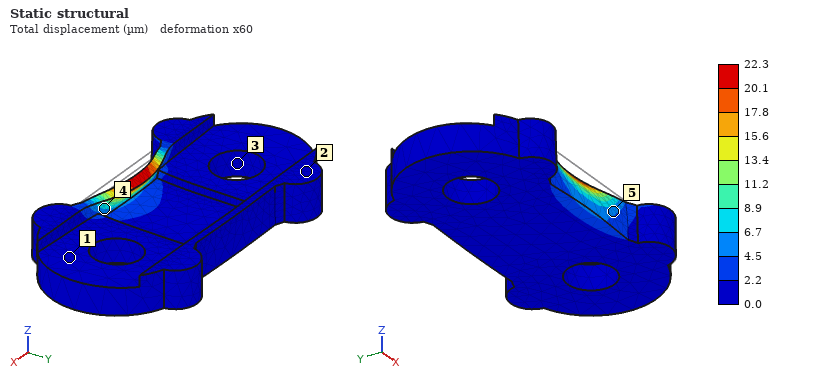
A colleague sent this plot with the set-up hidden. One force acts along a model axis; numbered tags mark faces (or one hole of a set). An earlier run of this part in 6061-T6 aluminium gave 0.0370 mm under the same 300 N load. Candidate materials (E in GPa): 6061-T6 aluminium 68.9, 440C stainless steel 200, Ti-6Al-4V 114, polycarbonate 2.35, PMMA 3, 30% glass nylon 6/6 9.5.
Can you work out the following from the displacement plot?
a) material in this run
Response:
Ti-6Al-4V
